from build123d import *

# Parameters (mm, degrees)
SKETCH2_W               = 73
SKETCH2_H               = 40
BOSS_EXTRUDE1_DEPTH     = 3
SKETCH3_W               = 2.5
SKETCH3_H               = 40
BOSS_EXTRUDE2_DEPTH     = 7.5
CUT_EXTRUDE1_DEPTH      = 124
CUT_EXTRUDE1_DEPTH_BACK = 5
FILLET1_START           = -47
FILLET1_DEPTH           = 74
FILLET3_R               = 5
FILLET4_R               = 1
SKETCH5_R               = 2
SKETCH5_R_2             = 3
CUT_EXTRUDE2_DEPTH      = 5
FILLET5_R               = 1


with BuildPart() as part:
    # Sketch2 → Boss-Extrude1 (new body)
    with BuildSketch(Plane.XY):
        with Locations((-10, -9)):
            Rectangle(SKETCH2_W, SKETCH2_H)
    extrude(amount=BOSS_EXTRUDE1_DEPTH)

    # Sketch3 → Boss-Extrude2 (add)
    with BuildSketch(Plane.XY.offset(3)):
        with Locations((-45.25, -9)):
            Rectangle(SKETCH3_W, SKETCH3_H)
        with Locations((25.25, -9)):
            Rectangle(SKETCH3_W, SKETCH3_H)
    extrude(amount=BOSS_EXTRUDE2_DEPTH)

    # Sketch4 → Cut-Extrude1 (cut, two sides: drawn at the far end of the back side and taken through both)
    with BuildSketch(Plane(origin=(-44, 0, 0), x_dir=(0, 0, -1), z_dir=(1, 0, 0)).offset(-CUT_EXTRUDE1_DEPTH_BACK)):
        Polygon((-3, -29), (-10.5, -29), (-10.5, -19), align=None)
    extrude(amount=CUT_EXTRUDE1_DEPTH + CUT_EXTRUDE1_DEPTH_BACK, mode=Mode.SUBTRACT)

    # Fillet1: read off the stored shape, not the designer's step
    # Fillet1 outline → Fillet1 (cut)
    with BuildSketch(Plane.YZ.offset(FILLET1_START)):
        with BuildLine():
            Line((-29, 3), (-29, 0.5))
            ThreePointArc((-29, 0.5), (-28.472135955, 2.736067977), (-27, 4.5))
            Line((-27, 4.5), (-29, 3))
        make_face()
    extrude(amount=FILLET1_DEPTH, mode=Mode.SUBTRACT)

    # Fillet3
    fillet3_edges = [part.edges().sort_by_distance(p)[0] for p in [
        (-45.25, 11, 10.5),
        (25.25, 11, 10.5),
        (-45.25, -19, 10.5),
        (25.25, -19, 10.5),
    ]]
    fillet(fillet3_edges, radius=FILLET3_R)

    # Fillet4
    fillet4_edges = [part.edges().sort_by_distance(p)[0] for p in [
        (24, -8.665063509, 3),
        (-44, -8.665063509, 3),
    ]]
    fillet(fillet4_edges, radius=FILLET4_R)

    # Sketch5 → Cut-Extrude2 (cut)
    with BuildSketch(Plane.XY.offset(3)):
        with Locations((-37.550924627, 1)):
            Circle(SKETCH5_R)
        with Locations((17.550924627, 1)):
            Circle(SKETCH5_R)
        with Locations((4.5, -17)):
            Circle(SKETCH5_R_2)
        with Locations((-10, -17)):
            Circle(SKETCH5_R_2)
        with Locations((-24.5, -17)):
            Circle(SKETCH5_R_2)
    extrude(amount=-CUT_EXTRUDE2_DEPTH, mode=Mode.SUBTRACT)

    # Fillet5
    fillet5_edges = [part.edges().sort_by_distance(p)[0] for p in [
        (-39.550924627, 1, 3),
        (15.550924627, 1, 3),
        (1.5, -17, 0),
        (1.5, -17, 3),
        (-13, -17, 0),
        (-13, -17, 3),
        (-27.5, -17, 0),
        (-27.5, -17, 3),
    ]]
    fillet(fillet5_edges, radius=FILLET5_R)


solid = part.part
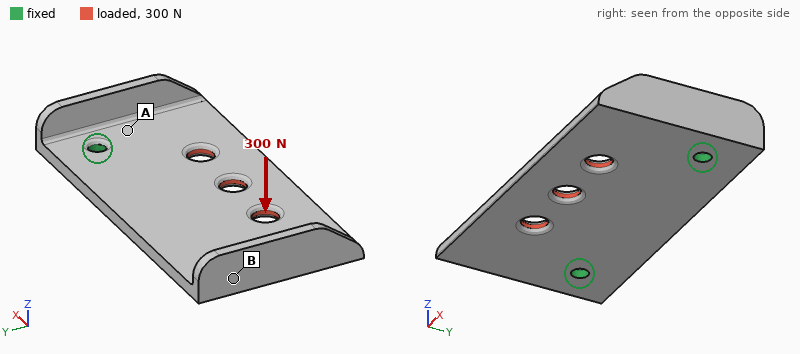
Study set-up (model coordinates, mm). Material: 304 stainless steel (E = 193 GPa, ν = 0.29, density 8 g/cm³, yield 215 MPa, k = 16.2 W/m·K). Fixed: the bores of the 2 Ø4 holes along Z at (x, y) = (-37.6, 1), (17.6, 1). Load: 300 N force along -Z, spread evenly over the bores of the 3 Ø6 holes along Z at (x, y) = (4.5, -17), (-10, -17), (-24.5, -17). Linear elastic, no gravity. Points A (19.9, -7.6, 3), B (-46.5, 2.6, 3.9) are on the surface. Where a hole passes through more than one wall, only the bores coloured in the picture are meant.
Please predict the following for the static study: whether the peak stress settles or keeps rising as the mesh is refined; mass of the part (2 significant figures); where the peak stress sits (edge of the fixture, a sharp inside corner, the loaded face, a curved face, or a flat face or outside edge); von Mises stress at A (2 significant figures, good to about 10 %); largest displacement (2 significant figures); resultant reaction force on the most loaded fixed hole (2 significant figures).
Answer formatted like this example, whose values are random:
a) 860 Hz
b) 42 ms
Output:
a) keeps rising
b) 77 g
c) edge of the fixture
d) 32 MPa
e) 72 µm
f) 150 N
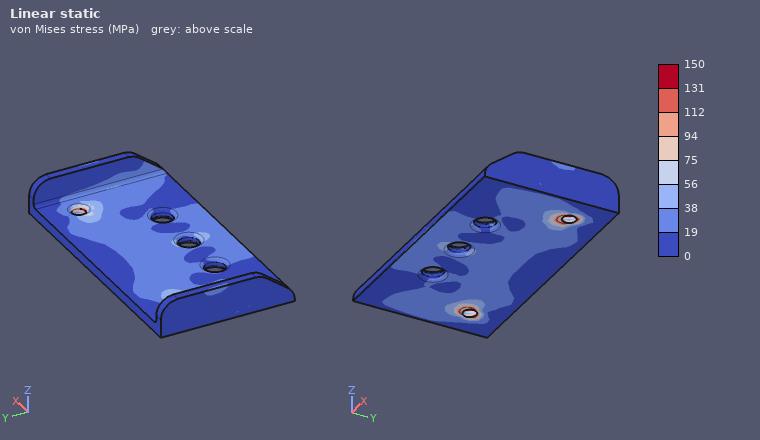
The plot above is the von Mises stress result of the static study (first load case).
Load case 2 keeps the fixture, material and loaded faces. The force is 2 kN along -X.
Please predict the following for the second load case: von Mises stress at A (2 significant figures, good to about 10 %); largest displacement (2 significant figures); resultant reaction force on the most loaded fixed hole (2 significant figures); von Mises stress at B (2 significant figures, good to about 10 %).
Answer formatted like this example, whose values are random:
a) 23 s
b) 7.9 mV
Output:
a) 10 MPa
b) 5.2 µm
c) 1.2 kN
d) 9.9 MPa
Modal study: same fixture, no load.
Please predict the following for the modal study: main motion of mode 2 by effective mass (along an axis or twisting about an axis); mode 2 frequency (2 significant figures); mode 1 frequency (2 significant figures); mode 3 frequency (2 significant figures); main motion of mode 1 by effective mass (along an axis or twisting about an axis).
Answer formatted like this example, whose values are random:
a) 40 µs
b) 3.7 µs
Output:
a) twisting about Y
b) 3700 Hz
c) 2300 Hz
d) 4300 Hz
e) along Z
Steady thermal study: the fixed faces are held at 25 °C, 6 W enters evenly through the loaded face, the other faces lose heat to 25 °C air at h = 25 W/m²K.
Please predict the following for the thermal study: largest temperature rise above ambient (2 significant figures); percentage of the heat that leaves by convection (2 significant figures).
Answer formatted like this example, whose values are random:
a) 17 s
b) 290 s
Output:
a) 44 K
b) 51 %
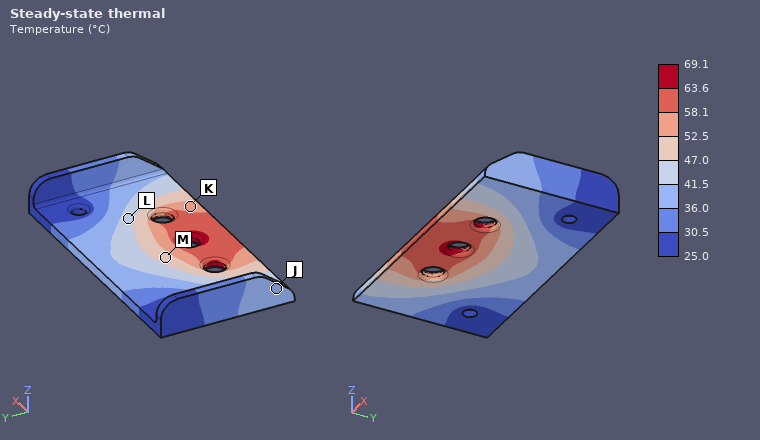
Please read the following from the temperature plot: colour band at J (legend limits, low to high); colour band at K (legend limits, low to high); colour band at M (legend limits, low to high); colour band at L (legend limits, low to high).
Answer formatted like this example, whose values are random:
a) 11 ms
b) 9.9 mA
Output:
a) 36.0 to 41.5 °C
b) 52.5 to 58.1 °C
c) 47.0 to 52.5 °C
d) 41.5 to 47.0 °C
